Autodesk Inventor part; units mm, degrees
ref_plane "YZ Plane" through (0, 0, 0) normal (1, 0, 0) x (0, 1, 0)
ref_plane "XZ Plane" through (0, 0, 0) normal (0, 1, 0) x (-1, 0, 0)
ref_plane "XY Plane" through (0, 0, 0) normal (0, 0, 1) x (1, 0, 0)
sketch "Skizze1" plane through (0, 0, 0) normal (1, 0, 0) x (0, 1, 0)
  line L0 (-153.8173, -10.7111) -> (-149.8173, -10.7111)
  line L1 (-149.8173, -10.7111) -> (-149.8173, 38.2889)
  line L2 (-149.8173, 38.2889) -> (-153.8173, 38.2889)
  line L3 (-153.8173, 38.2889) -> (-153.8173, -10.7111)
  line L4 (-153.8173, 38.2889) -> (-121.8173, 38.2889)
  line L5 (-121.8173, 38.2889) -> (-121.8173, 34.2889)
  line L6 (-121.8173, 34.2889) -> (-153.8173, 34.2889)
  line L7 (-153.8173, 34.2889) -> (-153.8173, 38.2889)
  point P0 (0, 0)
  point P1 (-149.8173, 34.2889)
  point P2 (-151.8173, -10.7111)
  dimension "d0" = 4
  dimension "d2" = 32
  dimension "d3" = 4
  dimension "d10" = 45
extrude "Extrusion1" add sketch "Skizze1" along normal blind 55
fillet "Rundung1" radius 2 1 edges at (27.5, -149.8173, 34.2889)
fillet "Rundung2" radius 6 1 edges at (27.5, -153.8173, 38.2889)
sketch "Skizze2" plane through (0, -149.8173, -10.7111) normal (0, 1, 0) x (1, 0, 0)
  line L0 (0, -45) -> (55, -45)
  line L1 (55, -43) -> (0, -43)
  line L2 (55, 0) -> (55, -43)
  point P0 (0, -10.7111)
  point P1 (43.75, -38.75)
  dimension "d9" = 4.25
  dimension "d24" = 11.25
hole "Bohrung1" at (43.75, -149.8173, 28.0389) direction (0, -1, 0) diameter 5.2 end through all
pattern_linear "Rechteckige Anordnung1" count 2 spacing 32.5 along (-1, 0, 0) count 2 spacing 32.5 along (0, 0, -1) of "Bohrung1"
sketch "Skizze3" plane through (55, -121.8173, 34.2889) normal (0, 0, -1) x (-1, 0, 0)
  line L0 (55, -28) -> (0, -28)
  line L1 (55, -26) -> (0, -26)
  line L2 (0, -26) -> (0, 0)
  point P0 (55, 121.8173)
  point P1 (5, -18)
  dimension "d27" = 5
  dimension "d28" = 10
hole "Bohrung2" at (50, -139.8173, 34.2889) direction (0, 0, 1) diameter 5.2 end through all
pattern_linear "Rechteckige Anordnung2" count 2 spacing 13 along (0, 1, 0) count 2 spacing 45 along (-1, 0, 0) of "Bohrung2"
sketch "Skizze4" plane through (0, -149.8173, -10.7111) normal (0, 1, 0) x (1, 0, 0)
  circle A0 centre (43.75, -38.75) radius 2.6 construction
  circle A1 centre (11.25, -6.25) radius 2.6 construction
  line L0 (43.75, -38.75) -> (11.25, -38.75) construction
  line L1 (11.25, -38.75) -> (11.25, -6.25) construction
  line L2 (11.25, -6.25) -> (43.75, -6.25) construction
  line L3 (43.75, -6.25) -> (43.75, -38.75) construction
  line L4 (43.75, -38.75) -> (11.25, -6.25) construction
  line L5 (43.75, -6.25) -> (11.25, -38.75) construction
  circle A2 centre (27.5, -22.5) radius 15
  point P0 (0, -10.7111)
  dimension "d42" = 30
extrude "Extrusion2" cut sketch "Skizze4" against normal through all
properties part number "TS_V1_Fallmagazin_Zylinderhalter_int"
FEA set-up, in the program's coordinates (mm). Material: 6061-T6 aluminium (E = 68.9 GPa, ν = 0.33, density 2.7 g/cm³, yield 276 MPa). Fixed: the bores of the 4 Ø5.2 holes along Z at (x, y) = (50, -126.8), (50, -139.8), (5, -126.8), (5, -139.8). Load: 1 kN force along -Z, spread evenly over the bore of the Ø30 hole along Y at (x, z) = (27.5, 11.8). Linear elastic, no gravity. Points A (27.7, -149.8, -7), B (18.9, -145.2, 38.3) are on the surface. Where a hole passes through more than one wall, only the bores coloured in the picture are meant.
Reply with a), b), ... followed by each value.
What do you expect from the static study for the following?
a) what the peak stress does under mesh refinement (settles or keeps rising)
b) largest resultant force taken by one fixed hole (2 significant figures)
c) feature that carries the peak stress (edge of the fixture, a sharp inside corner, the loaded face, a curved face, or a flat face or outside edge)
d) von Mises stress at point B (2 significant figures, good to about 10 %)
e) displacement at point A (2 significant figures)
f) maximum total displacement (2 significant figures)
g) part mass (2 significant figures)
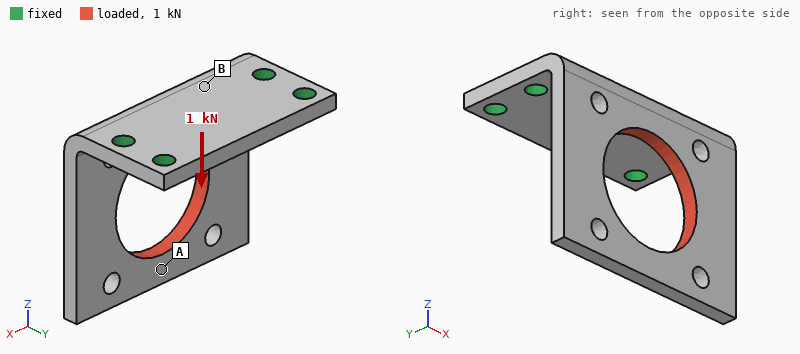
a) keeps rising
b) 610 N
c) edge of the fixture
d) 24 MPa
e) 0.16 mm
f) 0.18 mm
g) 35 g
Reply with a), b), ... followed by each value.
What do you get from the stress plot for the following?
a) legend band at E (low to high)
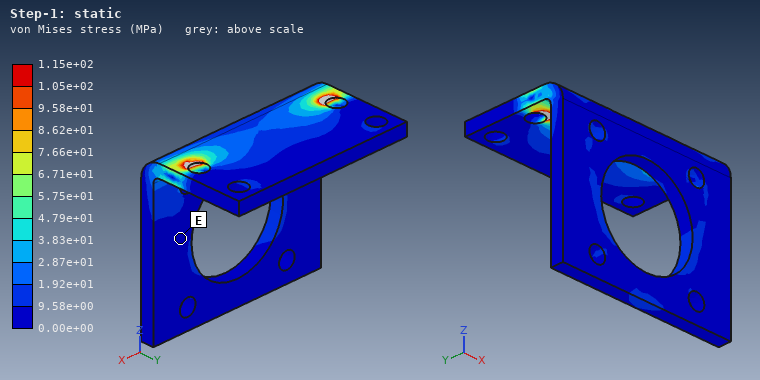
a) 0.00e+00 to 9.58e+00 MPa
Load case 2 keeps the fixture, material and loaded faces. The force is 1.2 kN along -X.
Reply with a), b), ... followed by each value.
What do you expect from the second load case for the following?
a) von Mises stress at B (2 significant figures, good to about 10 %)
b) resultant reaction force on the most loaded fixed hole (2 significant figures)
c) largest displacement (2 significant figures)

a) 14 MPa
b) 890 N
c) 0.15 mm
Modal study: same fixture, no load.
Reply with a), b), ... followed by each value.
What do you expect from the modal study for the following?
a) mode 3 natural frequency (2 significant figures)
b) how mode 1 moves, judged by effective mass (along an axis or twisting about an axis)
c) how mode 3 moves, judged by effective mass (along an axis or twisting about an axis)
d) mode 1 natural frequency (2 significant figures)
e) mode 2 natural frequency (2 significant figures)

a) 4500 Hz
b) along Y
c) along X
d) 1100 Hz
e) 2300 Hz
